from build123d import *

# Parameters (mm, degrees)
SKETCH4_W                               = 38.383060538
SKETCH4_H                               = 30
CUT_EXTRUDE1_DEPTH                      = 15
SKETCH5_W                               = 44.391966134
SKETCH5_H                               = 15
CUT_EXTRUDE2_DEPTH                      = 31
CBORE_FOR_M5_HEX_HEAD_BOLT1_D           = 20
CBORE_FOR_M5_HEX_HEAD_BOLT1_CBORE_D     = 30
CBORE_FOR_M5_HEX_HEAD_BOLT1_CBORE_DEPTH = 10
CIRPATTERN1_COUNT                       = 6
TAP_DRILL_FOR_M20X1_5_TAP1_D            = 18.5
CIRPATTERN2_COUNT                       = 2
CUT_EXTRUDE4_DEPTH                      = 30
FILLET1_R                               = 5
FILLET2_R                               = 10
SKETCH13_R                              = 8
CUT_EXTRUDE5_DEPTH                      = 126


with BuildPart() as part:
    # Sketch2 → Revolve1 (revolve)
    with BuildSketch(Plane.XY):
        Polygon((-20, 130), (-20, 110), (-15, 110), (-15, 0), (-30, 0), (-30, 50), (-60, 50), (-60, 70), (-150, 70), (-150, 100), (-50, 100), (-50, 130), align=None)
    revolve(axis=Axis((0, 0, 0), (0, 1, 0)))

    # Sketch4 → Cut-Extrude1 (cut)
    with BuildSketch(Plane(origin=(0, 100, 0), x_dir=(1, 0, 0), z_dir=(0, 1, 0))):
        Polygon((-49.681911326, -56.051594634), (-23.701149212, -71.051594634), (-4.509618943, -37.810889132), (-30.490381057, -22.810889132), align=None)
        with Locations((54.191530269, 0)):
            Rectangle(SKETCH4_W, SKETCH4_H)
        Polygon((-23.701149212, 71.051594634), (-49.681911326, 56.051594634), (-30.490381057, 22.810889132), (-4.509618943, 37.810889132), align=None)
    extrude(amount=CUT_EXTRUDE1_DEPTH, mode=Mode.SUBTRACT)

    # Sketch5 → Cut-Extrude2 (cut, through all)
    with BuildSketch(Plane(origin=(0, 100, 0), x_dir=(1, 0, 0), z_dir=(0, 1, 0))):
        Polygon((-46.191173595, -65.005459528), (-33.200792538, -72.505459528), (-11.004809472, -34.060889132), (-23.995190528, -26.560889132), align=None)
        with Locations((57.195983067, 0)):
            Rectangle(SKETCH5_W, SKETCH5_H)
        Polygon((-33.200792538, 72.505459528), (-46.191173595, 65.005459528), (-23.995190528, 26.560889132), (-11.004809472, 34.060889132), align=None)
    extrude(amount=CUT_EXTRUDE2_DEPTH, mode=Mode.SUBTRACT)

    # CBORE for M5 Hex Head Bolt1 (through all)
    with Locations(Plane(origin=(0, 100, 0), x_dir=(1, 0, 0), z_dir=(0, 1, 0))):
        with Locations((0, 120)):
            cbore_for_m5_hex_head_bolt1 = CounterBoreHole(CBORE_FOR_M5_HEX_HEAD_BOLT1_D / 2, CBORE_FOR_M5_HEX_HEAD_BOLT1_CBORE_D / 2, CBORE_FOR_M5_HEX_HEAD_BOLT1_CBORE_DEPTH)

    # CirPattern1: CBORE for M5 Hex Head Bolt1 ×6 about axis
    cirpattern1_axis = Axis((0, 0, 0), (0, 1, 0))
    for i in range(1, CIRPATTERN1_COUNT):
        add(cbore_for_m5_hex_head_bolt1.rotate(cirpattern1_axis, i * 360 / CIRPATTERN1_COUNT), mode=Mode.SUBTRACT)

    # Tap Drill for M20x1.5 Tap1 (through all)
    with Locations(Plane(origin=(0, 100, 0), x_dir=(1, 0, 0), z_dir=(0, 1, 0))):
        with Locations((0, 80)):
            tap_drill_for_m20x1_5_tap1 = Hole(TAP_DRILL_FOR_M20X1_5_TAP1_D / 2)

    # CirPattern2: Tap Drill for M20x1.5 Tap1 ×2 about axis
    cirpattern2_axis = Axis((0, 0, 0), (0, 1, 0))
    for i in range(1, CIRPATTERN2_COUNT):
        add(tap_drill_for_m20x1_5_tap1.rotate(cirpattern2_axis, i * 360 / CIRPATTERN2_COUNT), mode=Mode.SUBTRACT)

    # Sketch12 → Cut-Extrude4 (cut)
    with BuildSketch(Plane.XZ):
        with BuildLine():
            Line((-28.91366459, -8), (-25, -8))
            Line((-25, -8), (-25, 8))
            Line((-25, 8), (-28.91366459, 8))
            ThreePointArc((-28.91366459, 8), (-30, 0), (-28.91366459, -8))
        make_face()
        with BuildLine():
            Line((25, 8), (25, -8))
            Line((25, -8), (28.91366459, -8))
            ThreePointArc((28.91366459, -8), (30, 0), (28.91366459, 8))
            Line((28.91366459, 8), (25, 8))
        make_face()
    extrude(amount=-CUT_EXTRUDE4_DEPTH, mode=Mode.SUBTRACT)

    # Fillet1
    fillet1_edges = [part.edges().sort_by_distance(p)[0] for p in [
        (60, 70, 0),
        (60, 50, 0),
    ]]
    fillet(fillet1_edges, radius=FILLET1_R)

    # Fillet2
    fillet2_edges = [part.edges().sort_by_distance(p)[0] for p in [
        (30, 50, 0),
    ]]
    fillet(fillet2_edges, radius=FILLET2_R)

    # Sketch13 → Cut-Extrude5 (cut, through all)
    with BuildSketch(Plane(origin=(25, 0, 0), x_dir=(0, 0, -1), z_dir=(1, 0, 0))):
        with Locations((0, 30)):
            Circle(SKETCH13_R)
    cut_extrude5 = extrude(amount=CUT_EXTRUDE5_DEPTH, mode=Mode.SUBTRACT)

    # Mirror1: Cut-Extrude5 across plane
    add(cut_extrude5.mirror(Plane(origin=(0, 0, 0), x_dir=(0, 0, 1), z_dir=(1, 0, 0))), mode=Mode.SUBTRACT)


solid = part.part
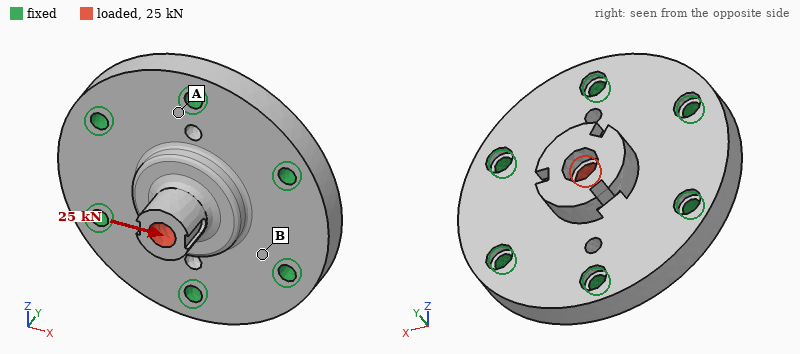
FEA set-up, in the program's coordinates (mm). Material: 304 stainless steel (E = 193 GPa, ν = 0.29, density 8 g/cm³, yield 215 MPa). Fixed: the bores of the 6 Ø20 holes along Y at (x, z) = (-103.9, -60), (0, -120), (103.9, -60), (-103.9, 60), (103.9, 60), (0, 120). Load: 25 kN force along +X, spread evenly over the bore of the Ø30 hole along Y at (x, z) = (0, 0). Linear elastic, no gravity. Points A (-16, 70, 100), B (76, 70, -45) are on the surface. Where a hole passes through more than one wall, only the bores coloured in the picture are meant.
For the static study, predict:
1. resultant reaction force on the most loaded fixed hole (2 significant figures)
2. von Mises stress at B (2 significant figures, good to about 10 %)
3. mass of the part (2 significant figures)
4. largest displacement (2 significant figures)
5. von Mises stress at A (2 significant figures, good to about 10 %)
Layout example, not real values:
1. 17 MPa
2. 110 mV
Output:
1. 5.5 kN
2. 5.5 MPa
3. 20 kg
4. 11 µm
5. 2.4 MPa
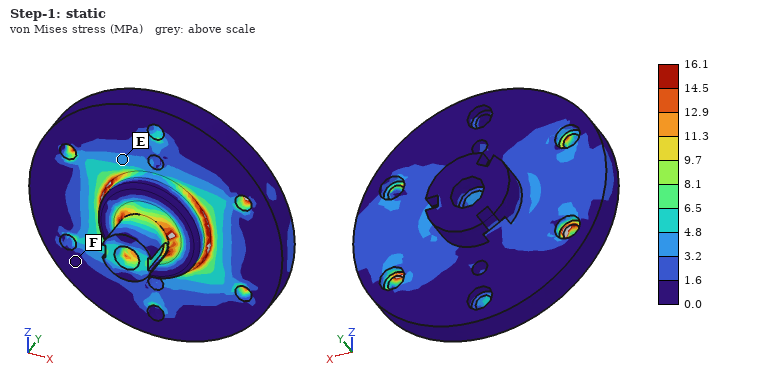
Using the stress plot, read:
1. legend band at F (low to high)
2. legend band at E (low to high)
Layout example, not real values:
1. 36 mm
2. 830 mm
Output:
1. 0.0 to 1.6 MPa
2. 3.2 to 4.8 MPa
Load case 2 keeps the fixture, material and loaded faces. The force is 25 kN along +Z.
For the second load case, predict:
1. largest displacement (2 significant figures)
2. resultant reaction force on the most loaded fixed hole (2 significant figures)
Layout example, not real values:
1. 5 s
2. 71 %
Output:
1. 12 µm
2. 5.7 kN
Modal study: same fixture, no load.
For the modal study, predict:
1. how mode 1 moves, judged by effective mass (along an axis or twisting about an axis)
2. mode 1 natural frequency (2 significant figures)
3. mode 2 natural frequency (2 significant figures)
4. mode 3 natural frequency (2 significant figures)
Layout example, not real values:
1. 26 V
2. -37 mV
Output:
1. along Y
2. 3100 Hz
3. 4800 Hz
4. 4900 Hz
